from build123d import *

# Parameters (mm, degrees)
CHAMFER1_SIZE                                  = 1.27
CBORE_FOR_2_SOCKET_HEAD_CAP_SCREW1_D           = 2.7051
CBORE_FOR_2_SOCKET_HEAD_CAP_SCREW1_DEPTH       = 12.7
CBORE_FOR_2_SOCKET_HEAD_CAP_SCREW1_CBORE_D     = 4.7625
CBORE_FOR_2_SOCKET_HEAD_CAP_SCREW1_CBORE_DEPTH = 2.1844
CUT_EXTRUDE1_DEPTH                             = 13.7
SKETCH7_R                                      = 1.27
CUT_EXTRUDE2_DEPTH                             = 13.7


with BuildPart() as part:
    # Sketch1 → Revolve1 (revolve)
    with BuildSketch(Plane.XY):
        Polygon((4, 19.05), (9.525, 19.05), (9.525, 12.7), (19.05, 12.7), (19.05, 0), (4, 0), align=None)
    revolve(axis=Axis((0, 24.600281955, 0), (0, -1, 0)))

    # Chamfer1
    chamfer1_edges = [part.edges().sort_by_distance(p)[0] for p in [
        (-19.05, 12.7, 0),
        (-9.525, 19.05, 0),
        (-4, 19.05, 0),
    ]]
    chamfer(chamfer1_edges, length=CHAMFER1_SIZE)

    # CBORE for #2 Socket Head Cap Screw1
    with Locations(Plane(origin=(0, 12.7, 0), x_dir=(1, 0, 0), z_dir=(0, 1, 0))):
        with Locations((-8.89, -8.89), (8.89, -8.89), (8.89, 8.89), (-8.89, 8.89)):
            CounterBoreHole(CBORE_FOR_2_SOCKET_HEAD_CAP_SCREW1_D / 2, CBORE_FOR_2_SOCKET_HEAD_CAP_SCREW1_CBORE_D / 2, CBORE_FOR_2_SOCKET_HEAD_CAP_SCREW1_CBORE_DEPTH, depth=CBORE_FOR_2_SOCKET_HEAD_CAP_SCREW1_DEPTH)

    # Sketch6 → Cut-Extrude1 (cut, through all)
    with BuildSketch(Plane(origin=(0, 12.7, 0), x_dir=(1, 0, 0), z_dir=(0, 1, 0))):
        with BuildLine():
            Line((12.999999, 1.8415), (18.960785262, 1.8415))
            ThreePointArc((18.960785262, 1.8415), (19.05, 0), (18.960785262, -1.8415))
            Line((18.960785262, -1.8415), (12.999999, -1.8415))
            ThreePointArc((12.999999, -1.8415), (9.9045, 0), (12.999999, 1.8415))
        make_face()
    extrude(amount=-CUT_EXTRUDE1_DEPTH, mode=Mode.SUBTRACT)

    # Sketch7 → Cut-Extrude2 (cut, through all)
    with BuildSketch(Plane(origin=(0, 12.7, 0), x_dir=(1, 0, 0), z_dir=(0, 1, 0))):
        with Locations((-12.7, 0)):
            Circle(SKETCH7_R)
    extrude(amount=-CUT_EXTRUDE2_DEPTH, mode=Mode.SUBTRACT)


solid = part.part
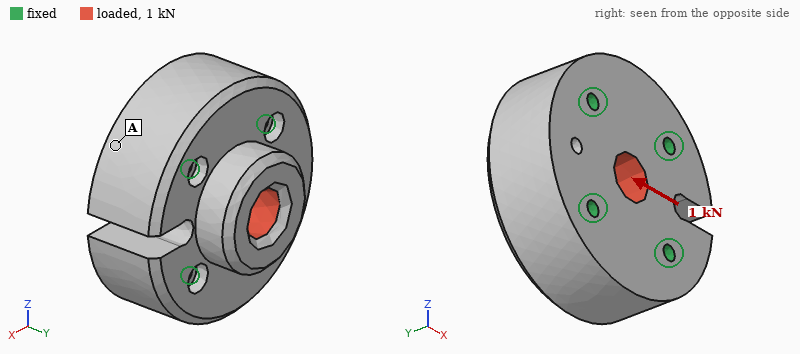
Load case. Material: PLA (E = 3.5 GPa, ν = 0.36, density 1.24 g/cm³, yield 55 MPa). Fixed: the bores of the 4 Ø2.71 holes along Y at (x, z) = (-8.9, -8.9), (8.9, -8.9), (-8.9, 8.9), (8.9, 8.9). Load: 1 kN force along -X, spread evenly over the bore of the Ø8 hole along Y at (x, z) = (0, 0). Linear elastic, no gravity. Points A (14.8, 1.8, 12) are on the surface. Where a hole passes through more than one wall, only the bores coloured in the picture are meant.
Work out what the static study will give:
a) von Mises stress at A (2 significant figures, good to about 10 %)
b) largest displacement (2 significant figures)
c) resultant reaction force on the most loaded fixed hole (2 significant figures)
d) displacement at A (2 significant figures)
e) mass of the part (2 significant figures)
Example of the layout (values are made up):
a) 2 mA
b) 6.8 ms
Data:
a) 1.1 MPa
b) 18 µm
c) 290 N
d) 3.8 µm
e) 18 g
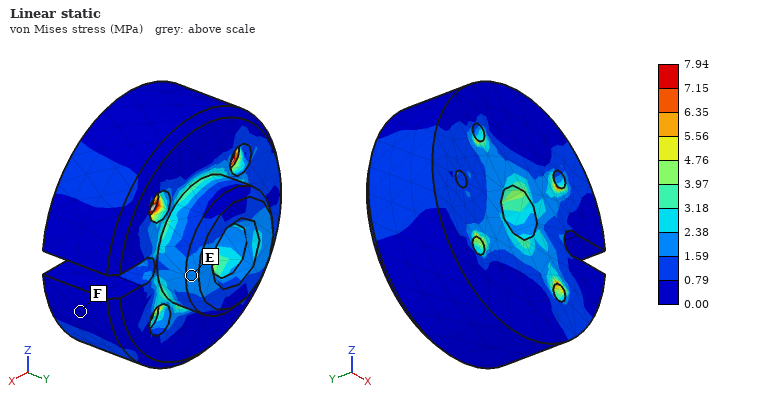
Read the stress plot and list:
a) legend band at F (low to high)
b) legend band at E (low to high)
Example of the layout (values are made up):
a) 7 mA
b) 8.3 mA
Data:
a) 0.00 to 0.79 MPa
b) 1.59 to 2.38 MPa
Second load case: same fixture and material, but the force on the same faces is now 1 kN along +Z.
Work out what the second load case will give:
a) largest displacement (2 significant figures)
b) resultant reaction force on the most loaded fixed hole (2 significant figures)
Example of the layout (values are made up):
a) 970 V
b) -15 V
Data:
a) 17 µm
b) 270 N
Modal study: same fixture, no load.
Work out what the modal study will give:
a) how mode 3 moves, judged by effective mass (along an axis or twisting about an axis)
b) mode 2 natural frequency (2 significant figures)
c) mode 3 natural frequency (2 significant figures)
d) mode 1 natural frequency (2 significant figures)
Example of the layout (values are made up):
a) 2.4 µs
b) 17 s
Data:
a) along Y
b) 15 kHz
c) 16 kHz
d) 15 kHz
